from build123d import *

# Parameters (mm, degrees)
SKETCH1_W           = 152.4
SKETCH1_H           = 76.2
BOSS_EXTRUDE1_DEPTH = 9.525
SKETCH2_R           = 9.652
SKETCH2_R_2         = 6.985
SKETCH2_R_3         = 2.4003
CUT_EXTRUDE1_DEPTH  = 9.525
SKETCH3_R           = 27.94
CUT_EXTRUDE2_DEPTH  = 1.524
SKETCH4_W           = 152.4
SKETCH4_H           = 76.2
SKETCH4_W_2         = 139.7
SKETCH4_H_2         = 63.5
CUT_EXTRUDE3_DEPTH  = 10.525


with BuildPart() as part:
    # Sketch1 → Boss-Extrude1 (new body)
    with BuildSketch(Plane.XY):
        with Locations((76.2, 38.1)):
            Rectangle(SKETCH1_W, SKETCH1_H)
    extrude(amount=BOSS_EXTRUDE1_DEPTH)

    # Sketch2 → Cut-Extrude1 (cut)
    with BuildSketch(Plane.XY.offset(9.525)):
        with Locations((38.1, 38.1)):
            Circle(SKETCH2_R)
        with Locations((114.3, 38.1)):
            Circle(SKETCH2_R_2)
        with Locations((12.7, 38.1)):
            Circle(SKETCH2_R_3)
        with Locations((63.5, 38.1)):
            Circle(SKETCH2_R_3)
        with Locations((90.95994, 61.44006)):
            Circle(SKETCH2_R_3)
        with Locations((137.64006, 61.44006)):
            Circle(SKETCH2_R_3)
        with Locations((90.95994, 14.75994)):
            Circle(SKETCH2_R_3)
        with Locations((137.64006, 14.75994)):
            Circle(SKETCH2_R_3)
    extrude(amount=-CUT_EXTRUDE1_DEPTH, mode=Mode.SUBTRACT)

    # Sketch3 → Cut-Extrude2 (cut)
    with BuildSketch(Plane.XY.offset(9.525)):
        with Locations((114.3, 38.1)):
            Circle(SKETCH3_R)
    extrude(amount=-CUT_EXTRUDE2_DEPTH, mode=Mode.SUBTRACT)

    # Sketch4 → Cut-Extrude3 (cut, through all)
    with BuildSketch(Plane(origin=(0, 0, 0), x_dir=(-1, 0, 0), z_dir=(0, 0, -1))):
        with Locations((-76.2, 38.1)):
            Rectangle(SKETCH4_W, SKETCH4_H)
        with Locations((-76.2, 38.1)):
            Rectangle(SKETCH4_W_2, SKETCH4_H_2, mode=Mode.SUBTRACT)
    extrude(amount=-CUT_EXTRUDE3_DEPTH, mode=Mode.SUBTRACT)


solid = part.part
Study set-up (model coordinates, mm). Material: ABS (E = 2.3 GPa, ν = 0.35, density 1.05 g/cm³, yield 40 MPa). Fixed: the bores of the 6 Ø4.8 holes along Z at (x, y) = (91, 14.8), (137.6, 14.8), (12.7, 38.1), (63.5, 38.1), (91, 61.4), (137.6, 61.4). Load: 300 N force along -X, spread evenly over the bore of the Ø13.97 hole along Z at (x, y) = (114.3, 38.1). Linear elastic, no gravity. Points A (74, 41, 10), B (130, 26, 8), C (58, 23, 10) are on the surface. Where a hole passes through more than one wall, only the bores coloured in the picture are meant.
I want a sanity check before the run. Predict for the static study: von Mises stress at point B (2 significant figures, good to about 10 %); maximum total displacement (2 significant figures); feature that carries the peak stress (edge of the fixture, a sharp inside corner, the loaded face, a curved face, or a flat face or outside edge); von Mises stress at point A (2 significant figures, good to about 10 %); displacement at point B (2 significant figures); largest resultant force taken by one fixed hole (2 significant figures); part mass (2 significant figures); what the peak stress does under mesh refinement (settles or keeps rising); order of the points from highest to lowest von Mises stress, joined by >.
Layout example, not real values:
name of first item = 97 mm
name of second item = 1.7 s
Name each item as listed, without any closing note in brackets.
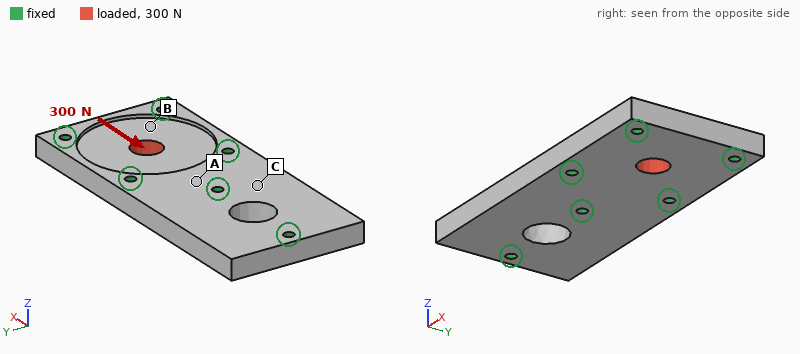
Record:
von Mises stress at point B = 0.62 MPa
maximum total displacement = 10 µm
feature that carries the peak stress = edge of the fixture
von Mises stress at point A = 0.25 MPa
displacement at point B = 4.7 µm
largest resultant force taken by one fixed hole = 70 N
part mass = 79 g
what the peak stress does under mesh refinement = keeps rising
order of the points from highest to lowest von Mises stress, joined by > = B > A > C
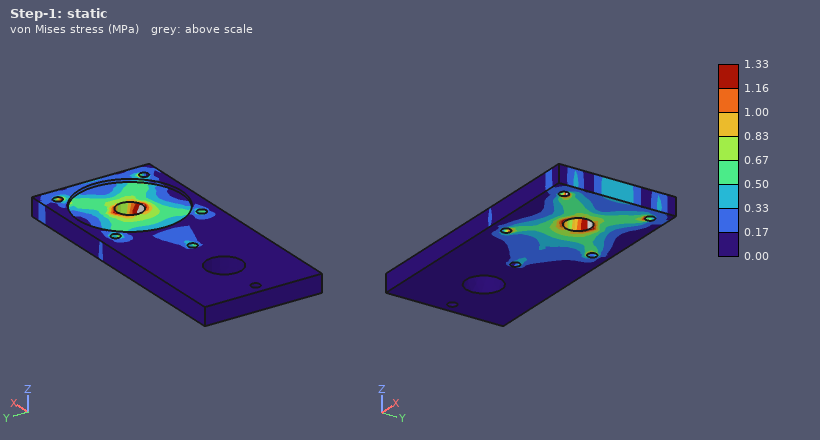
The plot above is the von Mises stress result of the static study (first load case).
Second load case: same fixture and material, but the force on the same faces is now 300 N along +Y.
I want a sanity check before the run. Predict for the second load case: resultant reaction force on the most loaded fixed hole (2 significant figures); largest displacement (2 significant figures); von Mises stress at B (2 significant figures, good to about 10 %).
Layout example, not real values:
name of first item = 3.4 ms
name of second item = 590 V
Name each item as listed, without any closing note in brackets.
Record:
resultant reaction force on the most loaded fixed hole = 82 N
largest displacement = 11 µm
von Mises stress at B = 0.66 MPa
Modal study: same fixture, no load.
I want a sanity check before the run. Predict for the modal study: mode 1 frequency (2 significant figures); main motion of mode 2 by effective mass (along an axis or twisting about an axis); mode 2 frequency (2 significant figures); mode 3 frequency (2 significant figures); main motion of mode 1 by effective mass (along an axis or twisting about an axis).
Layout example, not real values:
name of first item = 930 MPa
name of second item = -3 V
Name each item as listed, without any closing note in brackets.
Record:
mode 1 frequency = 1700 Hz
main motion of mode 2 by effective mass = along Z
mode 2 frequency = 2100 Hz
mode 3 frequency = 3500 Hz
main motion of mode 1 by effective mass = twisting about X
